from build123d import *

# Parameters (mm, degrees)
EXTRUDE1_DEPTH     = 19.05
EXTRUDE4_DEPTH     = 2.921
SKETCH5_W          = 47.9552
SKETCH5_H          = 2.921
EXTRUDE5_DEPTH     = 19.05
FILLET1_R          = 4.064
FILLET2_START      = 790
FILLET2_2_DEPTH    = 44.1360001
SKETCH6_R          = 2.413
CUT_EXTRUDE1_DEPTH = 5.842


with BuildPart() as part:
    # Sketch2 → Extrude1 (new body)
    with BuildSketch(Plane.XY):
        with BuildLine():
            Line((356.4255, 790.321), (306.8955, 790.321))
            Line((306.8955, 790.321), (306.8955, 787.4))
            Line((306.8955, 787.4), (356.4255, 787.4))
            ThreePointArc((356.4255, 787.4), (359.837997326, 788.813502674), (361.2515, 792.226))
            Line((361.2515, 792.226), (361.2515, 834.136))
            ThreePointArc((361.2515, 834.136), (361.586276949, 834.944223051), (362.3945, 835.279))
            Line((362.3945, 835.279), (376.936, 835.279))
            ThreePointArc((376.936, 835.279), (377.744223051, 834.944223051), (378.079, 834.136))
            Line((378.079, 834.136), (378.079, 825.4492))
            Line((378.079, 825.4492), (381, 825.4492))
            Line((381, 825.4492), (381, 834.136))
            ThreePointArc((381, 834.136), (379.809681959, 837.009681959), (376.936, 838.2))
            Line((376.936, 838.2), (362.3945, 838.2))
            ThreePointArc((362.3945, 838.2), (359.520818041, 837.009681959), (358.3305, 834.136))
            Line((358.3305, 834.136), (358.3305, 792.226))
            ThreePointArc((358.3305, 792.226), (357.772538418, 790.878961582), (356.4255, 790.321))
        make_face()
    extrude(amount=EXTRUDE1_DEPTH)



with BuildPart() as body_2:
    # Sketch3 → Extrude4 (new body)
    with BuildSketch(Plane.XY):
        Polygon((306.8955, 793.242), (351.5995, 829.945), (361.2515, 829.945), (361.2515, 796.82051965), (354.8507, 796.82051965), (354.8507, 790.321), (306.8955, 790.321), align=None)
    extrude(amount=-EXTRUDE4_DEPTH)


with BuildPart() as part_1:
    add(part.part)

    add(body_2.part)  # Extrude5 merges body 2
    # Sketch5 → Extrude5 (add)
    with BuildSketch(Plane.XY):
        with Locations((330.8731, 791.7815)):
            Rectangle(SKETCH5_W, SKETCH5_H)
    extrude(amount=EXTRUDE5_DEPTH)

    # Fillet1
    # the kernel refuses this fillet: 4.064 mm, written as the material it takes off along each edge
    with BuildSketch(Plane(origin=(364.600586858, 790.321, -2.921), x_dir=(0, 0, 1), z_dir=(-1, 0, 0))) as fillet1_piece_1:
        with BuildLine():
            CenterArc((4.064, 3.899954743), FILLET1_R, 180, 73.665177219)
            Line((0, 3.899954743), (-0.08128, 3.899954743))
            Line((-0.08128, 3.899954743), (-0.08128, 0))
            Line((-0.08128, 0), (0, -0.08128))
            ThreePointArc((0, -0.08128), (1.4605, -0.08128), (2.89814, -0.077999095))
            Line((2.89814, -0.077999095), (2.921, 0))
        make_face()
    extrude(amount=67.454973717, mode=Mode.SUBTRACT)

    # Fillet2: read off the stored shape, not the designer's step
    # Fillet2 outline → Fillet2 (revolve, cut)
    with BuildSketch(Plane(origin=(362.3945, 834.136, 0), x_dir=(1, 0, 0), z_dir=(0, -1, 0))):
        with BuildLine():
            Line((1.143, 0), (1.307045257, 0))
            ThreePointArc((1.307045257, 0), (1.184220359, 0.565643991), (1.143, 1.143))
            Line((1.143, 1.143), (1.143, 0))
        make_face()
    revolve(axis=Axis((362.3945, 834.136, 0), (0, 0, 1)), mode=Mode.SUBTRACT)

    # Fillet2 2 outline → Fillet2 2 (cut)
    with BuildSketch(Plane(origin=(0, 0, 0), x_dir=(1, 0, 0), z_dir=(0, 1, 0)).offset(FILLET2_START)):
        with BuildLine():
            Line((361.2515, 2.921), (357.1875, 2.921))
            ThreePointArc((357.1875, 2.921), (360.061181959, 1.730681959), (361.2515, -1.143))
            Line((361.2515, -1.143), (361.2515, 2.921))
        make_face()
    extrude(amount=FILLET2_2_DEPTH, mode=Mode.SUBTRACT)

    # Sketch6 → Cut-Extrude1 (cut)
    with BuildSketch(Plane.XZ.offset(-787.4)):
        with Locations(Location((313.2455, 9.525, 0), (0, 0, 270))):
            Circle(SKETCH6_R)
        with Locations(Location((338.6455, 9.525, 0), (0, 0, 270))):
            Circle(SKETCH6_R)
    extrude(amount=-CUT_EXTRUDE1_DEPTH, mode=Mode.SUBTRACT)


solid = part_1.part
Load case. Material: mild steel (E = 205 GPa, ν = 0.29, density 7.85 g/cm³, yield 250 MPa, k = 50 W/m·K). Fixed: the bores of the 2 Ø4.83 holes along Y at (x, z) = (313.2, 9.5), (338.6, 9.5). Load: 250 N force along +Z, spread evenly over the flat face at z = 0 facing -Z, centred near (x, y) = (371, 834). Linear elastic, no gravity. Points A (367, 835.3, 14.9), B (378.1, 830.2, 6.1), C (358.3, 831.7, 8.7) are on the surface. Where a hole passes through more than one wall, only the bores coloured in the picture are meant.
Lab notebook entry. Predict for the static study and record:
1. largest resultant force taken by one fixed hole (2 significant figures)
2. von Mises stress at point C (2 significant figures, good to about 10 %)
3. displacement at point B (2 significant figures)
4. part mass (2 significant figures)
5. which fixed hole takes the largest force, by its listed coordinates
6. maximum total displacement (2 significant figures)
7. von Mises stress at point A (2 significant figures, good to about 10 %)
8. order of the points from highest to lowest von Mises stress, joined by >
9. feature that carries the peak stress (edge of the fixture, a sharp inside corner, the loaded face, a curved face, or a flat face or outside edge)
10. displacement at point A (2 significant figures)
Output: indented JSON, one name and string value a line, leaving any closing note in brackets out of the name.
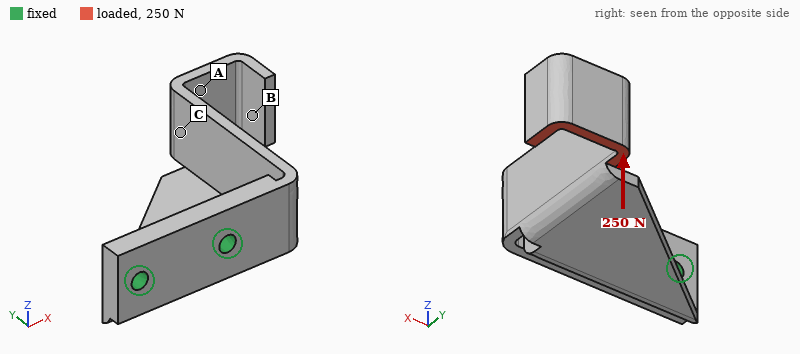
{
  "largest resultant force taken by one fixed hole": "480 N",
  "von Mises stress at point C": "67 MPa",
  "displacement at point B": "0.25 mm",
  "part mass": "100 g",
  "which fixed hole takes the largest force, by its listed coordinates": "(338.6, 9.5)",
  "maximum total displacement": "0.30 mm",
  "von Mises stress at point A": "34 MPa",
  "order of the points from highest to lowest von Mises stress, joined by >": "C > A > B",
  "feature that carries the peak stress": "a curved face",
  "displacement at point A": "0.21 mm"
}
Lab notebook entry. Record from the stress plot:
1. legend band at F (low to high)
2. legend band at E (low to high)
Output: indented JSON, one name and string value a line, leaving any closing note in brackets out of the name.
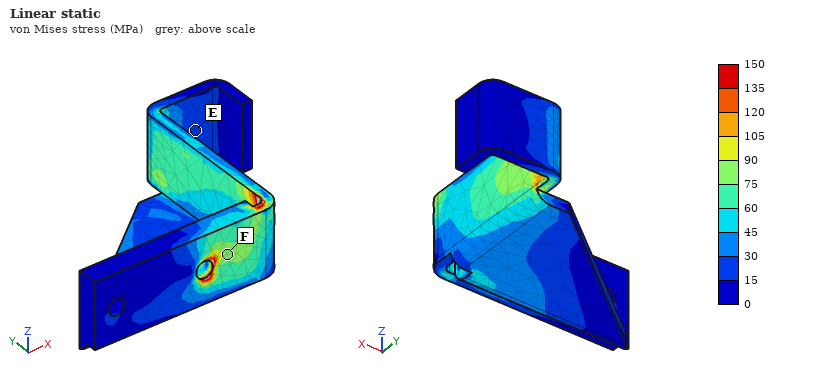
{
  "legend band at F": "75 to 90 MPa",
  "legend band at E": "15 to 30 MPa"
}
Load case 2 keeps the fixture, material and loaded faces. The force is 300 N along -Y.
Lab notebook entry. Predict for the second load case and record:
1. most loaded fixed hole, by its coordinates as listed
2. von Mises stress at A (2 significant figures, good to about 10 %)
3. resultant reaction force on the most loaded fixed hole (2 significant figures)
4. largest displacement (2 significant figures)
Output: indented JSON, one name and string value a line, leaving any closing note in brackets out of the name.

{
  "most loaded fixed hole, by its coordinates as listed": "(338.6, 9.5)",
  "von Mises stress at A": "76 MPa",
  "resultant reaction force on the most loaded fixed hole": "580 N",
  "largest displacement": "0.22 mm"
}
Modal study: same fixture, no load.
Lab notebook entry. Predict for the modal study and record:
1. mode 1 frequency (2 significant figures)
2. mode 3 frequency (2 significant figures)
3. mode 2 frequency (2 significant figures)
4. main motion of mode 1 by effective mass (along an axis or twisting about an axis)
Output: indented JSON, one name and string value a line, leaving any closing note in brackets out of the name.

{
  "mode 1 frequency": "1100 Hz",
  "mode 3 frequency": "2300 Hz",
  "mode 2 frequency": "1700 Hz",
  "main motion of mode 1 by effective mass": "along Z"
}
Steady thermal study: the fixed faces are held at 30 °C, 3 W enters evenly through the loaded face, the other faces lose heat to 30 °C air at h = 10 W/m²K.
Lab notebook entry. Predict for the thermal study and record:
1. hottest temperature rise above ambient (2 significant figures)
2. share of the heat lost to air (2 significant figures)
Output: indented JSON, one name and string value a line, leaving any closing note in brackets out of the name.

{
  "hottest temperature rise above ambient": "42 K",
  "share of the heat lost to air": "30 %"
}
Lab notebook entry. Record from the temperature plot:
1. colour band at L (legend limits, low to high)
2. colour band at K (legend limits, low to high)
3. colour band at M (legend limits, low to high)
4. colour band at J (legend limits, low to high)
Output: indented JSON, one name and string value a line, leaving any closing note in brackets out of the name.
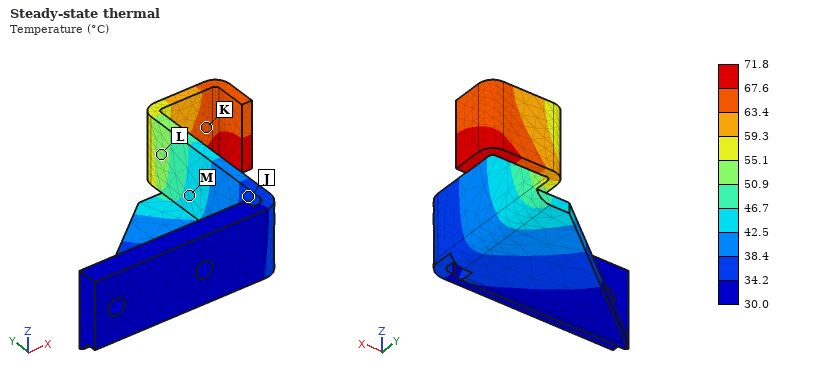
{
  "colour band at L": "50.9 to 55.1 °C",
  "colour band at K": "63.4 to 67.6 °C",
  "colour band at M": "42.5 to 46.7 °C",
  "colour band at J": "34.2 to 38.4 °C"
}
